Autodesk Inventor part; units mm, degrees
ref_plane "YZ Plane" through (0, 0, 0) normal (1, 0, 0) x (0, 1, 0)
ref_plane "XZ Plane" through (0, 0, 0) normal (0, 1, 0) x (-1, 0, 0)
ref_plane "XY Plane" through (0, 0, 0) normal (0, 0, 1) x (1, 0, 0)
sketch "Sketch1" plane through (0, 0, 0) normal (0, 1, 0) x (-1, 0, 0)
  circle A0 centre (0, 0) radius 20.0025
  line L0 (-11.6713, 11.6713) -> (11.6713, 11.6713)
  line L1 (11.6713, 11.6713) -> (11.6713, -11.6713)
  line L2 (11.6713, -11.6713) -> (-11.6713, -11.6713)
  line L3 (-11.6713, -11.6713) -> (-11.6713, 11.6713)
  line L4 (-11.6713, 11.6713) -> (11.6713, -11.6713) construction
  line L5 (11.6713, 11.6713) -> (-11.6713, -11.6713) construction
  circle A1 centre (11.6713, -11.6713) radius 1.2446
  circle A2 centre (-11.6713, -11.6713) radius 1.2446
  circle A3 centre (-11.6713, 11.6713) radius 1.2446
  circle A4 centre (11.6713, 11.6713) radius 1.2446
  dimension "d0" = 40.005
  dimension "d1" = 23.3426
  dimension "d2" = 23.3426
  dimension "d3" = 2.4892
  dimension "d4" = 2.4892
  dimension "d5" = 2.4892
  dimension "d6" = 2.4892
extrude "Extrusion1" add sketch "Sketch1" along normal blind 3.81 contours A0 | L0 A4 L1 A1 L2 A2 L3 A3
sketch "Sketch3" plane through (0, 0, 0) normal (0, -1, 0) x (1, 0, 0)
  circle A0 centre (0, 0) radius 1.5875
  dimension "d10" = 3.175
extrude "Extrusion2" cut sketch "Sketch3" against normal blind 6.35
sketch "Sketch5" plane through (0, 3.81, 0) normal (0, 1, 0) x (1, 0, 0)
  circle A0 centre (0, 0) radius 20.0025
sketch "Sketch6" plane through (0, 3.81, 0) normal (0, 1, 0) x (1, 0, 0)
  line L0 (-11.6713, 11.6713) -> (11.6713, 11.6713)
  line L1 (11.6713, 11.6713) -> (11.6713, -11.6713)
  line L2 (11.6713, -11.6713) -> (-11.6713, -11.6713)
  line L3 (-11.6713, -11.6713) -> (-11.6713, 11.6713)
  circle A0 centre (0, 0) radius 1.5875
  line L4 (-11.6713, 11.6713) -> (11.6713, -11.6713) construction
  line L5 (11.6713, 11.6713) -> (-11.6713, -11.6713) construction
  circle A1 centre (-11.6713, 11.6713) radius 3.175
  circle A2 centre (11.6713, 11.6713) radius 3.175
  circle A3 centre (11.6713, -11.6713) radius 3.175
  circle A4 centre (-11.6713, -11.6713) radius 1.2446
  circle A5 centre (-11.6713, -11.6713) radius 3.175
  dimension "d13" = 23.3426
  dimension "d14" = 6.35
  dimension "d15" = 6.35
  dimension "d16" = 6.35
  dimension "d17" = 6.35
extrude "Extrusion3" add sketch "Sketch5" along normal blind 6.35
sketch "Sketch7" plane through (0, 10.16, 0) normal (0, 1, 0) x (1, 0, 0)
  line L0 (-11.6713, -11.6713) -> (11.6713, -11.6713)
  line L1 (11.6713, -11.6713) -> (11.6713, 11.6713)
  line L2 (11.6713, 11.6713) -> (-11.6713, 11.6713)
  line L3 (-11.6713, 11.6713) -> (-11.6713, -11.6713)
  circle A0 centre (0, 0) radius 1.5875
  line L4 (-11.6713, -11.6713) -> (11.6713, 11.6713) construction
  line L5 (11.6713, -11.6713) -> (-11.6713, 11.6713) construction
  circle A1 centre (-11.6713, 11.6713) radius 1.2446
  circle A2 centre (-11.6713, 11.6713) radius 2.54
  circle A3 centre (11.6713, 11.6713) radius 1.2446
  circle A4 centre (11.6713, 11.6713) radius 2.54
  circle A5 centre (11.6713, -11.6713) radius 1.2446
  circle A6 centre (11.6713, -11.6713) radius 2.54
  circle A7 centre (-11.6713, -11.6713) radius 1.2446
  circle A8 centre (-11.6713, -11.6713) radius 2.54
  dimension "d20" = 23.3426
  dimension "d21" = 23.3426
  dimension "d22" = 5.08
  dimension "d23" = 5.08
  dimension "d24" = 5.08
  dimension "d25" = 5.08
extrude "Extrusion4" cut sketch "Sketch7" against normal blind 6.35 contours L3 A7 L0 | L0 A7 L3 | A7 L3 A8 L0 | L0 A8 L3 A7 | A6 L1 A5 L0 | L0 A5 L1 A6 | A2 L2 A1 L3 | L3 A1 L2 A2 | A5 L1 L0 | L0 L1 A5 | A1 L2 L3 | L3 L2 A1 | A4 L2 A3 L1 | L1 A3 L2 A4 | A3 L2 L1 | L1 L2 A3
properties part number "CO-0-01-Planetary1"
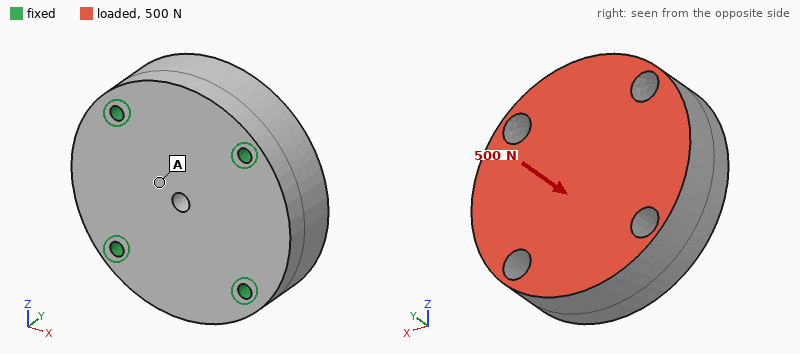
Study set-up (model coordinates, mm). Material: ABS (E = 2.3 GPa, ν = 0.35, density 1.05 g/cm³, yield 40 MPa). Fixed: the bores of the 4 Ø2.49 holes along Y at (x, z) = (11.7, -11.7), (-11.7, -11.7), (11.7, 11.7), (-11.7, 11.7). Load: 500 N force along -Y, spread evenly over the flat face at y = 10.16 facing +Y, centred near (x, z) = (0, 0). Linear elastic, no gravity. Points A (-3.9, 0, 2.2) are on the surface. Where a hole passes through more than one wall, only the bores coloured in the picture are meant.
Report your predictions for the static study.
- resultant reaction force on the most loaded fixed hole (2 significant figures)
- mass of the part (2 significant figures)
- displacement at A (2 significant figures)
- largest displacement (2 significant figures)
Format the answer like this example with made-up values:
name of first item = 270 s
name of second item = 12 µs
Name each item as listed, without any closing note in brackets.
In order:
resultant reaction force on the most loaded fixed hole = 130 N
mass of the part = 13 g
displacement at A = 18 µm
largest displacement = 19 µm
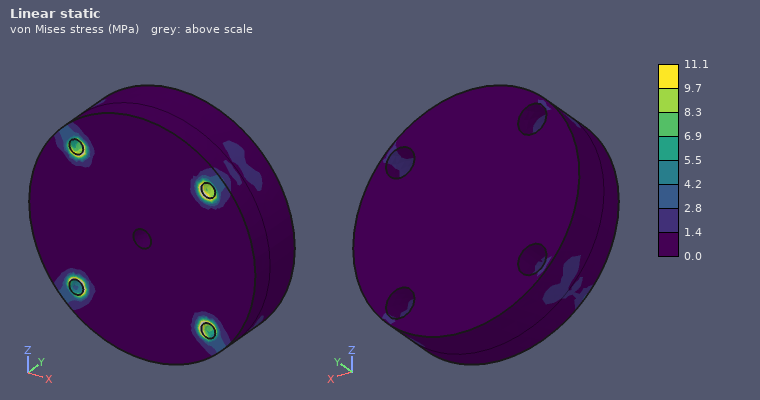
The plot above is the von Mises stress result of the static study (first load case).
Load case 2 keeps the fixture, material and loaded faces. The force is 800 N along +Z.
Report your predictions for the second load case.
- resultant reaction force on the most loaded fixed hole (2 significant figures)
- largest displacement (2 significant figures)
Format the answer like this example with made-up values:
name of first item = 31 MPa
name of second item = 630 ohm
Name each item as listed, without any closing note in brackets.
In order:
resultant reaction force on the most loaded fixed hole = 240 N
largest displacement = 55 µm
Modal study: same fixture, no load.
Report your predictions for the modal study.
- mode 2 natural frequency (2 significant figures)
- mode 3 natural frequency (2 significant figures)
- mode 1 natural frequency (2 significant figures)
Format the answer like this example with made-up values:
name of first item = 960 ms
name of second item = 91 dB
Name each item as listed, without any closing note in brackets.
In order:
mode 2 natural frequency = 8400 Hz
mode 3 natural frequency = 8400 Hz
mode 1 natural frequency = 8100 Hz
